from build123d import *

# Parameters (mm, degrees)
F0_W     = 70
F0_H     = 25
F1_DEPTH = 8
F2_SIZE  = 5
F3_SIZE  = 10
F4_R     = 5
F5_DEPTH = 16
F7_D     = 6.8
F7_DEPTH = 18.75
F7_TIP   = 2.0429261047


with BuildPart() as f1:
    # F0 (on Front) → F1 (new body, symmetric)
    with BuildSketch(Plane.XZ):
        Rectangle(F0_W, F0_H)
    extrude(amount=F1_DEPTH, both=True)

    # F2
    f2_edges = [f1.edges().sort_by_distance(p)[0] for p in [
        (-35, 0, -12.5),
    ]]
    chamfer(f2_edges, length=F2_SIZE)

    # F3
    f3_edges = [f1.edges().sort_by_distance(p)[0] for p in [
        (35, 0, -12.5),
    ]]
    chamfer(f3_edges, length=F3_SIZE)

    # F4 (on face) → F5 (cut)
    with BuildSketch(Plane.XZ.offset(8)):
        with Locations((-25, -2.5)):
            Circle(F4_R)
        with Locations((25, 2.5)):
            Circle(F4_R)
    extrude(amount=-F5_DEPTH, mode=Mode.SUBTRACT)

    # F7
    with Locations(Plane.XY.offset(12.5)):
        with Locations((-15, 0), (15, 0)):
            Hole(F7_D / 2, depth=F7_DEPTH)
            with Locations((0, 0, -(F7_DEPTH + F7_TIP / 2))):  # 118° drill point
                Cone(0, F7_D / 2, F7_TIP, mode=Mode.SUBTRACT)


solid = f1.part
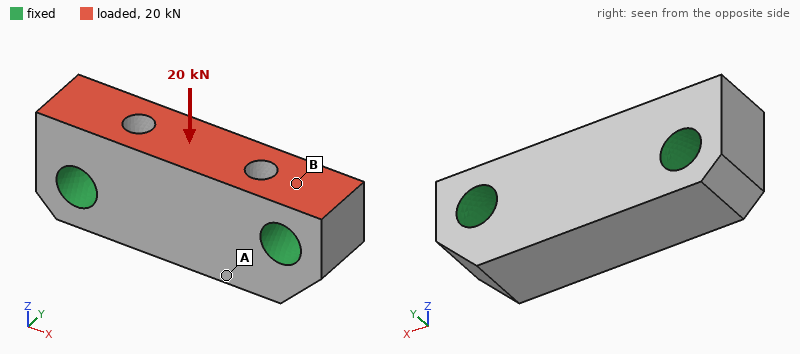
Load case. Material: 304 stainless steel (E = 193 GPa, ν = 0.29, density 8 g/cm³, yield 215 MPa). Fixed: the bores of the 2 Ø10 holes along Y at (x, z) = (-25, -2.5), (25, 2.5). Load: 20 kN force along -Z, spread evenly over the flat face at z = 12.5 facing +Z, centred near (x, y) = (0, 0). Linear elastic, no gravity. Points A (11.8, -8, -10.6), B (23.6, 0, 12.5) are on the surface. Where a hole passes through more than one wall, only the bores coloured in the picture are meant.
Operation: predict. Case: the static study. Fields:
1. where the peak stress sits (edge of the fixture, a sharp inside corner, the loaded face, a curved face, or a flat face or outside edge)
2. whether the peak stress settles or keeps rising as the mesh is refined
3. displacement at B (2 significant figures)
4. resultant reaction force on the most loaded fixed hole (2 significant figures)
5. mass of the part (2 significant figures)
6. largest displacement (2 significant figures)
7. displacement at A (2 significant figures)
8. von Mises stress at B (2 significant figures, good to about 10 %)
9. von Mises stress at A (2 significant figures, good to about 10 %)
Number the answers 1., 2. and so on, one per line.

1. edge of the fixture
2. keeps rising
3. 0.87 µm
4. 10 kN
5. 180 g
6. 5.8 µm
7. 3.4 µm
8. 37 MPa
9. 15 MPa
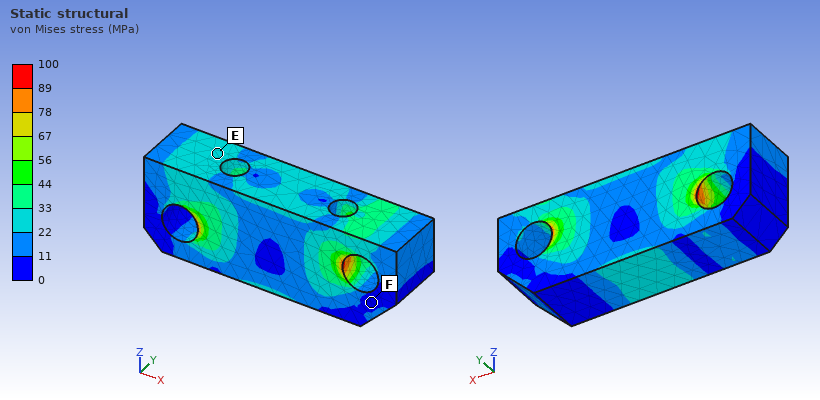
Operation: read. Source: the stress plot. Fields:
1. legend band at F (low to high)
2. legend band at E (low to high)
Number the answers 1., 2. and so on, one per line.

1. 0 to 11 MPa
2. 22 to 33 MPa
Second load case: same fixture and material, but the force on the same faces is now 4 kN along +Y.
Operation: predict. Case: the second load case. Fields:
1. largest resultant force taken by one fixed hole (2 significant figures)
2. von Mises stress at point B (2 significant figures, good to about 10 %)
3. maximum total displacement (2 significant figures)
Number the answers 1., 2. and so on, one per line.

1. 2.0 kN
2. 12 MPa
3. 4.6 µm
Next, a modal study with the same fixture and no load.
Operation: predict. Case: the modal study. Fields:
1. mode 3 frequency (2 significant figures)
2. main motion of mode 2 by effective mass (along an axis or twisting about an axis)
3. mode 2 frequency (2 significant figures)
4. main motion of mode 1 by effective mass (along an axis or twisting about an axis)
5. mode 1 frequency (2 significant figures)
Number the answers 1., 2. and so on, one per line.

1. 26 kHz
2. along Z
3. 23 kHz
4. along Y
5. 20 kHz
